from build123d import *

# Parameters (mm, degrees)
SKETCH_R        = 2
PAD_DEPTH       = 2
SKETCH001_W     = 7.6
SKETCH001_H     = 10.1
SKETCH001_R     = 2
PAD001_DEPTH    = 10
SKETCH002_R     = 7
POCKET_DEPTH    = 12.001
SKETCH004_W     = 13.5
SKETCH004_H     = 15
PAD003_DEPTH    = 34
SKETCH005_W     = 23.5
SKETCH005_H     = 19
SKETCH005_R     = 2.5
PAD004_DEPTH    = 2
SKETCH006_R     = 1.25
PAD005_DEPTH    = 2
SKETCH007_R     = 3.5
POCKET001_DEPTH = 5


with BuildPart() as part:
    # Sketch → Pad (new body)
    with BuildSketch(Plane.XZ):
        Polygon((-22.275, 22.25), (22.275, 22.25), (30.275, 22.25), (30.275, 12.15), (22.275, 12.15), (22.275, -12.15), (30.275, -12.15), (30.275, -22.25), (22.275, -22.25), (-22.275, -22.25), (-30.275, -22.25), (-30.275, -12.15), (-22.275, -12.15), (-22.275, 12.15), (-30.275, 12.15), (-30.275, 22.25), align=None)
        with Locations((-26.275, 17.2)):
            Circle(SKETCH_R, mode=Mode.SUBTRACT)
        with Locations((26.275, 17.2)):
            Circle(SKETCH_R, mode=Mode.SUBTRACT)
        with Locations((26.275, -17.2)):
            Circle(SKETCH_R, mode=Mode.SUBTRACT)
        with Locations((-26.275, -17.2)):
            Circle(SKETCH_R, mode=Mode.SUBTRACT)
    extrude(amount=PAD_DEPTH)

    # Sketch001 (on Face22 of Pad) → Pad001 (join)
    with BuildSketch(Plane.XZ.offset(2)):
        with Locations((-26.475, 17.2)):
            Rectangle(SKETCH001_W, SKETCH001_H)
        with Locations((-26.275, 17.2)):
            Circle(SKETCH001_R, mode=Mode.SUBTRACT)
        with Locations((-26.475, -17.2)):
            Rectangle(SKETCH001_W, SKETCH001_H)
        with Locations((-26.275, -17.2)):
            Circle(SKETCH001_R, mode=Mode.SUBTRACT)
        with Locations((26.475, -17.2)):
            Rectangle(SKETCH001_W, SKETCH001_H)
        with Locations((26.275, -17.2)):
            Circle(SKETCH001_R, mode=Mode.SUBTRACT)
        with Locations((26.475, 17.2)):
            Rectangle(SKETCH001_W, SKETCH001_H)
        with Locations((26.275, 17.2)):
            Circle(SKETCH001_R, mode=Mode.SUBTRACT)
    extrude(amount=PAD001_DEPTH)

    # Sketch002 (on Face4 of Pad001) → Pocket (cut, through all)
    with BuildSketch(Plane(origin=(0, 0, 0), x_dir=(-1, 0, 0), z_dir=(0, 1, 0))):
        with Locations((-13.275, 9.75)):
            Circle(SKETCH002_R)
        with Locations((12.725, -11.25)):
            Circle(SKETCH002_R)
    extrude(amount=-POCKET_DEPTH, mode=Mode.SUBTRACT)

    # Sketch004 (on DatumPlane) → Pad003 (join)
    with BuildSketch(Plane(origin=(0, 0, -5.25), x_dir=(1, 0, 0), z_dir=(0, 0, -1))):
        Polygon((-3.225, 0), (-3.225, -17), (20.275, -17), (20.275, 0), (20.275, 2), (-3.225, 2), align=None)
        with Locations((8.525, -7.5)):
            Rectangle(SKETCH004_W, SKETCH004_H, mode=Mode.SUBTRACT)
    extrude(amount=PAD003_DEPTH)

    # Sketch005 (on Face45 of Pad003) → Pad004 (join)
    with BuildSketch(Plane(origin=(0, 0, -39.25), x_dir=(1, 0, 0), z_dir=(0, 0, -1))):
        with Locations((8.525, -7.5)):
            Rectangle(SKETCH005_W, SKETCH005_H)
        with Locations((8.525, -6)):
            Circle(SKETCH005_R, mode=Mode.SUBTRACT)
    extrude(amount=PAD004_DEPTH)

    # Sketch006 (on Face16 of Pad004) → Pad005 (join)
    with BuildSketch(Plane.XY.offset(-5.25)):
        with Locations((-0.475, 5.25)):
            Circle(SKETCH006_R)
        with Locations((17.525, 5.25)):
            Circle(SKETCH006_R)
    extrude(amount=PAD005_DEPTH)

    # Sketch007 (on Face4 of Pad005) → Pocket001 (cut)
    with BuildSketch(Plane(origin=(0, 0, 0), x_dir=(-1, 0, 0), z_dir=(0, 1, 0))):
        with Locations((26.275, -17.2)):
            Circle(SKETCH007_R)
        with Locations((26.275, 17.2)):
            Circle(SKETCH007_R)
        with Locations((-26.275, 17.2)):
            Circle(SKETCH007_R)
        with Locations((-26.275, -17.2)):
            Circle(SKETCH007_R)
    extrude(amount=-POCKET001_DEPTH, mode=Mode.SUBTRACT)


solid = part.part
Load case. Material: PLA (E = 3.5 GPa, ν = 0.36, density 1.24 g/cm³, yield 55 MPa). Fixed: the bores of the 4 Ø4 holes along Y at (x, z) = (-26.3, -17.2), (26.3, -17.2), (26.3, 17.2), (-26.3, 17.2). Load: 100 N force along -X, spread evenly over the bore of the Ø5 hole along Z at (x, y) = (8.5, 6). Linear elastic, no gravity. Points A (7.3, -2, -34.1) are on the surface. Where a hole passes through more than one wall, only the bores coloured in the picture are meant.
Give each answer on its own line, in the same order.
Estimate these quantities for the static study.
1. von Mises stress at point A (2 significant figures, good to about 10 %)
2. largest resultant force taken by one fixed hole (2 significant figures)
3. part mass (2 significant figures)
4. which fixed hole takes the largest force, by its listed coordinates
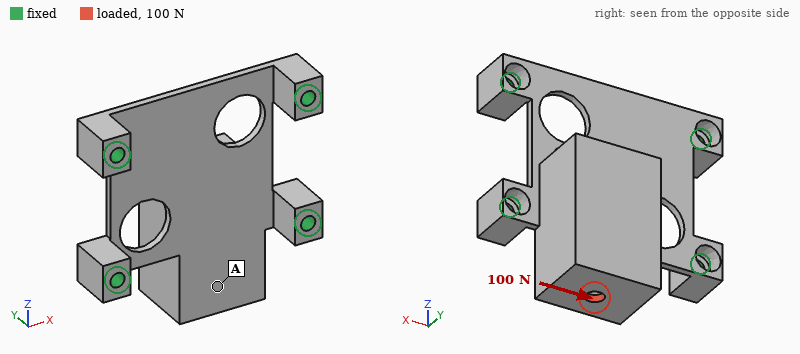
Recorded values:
2.8 MPa
73 N
18 g
(26.3, -17.2)
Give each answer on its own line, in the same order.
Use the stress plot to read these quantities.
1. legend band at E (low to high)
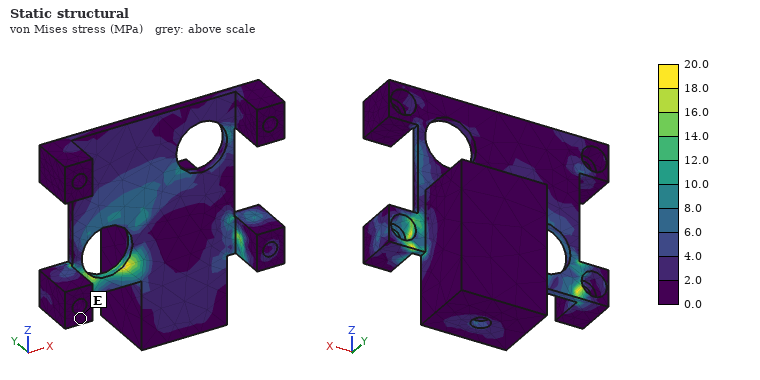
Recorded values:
0.0 to 2.0 MPa
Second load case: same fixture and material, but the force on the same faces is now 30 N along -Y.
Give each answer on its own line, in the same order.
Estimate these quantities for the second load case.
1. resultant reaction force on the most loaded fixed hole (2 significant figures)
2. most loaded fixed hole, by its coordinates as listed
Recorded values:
32 N
(26.3, -17.2)
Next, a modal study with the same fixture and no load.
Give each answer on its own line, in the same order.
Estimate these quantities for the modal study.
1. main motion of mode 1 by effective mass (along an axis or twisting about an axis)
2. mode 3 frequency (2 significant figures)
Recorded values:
along Y
1700 Hz
